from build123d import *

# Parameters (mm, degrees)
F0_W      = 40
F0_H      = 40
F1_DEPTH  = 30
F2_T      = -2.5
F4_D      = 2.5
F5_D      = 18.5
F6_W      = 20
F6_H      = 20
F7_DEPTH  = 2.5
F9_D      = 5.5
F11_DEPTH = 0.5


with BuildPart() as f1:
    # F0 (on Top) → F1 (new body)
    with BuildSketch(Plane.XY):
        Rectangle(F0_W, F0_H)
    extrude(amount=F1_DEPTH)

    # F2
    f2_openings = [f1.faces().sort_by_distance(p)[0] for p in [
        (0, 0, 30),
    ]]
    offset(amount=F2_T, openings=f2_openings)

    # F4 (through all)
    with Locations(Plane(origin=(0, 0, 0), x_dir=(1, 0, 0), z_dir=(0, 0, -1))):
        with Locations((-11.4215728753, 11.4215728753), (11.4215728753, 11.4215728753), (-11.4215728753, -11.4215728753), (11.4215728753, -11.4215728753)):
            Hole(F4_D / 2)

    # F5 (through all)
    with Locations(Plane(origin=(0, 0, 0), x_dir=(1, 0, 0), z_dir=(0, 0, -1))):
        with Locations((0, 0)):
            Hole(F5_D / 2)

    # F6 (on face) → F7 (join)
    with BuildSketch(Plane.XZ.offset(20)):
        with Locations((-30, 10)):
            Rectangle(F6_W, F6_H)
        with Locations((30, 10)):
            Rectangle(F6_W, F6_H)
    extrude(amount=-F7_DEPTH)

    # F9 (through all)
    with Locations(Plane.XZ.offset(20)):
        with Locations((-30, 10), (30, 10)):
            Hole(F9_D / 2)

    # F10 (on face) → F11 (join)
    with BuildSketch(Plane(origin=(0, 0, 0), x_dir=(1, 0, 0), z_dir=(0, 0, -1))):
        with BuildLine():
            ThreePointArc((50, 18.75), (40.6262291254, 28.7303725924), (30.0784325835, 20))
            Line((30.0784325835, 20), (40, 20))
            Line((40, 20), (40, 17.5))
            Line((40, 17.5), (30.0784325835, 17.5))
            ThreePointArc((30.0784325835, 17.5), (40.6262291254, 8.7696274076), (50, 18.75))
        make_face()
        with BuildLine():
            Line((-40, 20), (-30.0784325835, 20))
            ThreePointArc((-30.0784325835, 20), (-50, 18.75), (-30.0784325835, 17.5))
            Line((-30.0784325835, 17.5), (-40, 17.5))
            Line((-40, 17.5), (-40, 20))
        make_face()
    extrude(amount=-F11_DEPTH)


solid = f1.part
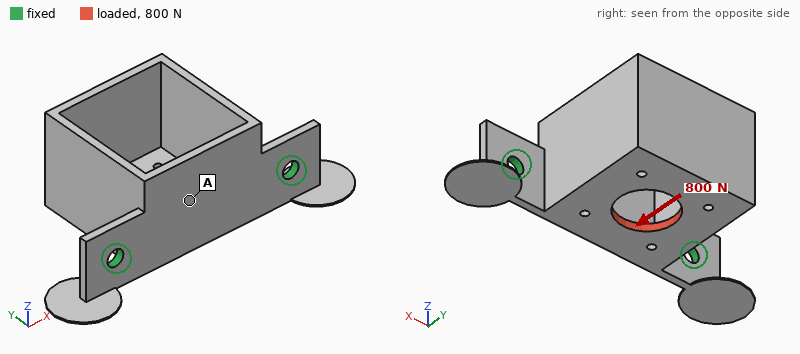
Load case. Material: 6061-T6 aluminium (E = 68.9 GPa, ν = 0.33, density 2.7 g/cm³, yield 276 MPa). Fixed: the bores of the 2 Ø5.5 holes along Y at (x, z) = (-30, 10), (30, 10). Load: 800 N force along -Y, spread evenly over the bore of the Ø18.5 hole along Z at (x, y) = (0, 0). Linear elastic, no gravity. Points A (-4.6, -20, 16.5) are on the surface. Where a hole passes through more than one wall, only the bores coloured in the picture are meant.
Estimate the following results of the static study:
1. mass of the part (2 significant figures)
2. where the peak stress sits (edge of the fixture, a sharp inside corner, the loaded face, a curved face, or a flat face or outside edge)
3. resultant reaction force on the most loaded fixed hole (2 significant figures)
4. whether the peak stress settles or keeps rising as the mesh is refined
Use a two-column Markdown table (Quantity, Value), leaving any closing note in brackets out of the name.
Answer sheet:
| Quantity | Value |
|---|---|
| mass of the part | 43 g |
| where the peak stress sits | edge of the fixture |
| resultant reaction force on the most loaded fixed hole | 450 N |
| whether the peak stress settles or keeps rising as the mesh is refined | keeps rising |
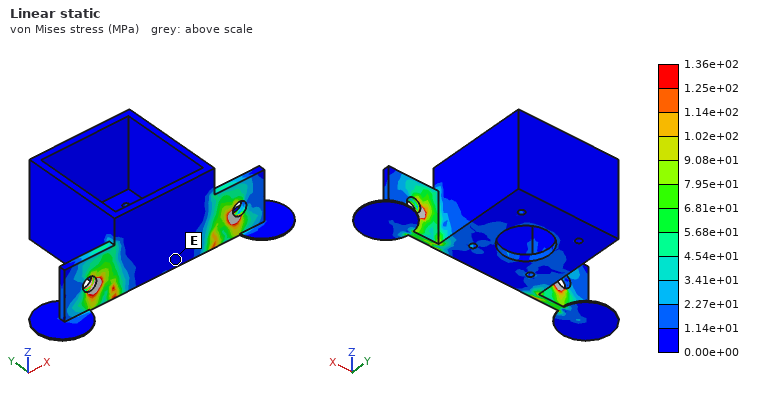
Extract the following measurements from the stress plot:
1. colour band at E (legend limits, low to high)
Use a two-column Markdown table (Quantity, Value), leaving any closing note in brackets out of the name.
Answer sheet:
| Quantity | Value |
|---|---|
| colour band at E | 0.00e+00 to 1.14e+01 MPa |
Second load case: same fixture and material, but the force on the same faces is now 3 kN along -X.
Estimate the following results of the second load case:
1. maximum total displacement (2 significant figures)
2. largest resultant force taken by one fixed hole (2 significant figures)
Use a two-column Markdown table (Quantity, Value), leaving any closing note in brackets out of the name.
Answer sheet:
| Quantity | Value |
|---|---|
| maximum total displacement | 0.38 mm |
| largest resultant force taken by one fixed hole | 2.0 kN |
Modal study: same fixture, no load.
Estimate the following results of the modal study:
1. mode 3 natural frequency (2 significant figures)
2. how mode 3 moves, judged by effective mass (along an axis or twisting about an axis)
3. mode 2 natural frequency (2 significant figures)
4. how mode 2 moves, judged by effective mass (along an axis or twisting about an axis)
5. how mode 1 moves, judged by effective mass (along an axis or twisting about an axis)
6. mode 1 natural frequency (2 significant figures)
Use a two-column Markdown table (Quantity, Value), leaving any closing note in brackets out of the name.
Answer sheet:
| Quantity | Value |
|---|---|
| mode 3 natural frequency | 3900 Hz |
| how mode 3 moves, judged by effective mass | along Y |
| mode 2 natural frequency | 1900 Hz |
| how mode 2 moves, judged by effective mass | along X |
| how mode 1 moves, judged by effective mass | along Z |
| mode 1 natural frequency | 960 Hz |
